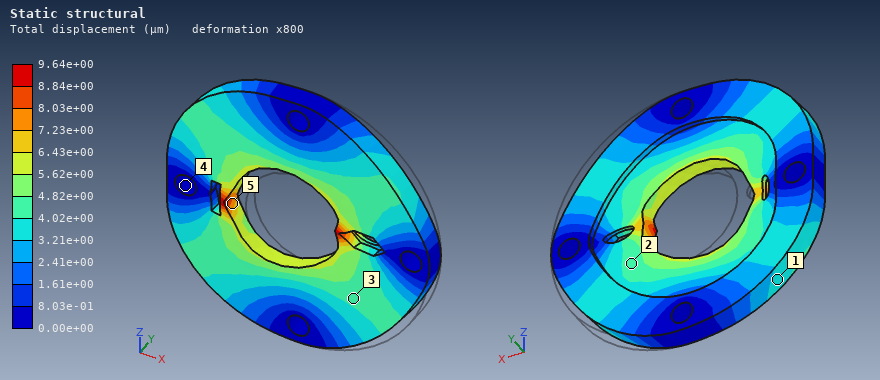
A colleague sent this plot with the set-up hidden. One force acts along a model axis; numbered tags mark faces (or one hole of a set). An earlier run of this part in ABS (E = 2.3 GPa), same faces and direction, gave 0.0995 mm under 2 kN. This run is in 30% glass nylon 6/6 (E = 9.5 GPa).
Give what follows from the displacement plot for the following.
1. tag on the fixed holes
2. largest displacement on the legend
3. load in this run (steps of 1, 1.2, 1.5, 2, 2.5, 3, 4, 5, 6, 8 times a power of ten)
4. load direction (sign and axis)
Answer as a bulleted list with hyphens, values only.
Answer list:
- 4
- 9.64e+00 µm
- 800 N
- -X
